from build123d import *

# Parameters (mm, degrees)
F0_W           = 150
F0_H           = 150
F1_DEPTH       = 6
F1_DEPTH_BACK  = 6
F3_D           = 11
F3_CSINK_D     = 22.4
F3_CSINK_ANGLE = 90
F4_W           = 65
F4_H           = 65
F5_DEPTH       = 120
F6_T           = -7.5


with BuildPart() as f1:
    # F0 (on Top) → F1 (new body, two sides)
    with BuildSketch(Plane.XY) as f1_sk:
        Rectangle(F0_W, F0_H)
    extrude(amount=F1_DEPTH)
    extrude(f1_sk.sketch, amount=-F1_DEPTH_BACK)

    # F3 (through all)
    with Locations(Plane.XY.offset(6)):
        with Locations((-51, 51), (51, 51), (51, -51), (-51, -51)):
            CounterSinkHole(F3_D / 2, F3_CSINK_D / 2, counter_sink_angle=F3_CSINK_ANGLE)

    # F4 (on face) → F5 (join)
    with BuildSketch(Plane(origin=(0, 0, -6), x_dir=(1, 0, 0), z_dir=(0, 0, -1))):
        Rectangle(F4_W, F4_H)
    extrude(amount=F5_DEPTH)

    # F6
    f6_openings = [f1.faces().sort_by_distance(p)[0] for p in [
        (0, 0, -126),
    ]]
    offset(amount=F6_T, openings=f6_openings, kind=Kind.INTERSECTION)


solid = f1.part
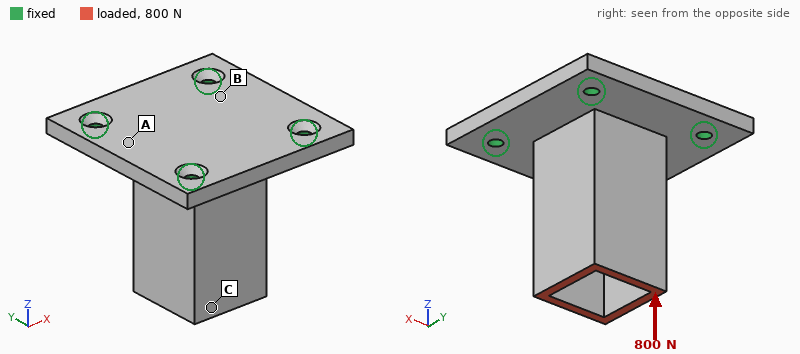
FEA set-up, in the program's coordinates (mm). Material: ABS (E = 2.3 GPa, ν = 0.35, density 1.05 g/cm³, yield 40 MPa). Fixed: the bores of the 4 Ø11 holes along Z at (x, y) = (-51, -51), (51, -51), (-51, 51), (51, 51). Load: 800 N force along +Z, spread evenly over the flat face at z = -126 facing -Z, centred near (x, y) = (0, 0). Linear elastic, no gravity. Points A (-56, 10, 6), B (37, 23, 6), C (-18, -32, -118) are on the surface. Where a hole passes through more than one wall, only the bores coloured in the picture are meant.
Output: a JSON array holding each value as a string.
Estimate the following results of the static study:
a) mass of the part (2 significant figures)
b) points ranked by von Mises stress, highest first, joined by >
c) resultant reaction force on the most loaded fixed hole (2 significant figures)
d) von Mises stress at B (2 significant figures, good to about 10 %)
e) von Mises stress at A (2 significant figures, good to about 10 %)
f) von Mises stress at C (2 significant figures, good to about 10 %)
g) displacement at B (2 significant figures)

["480 g", "B > A > C", "240 N", "1.6 MPa", "0.97 MPa", "0.46 MPa", "0.086 mm"]
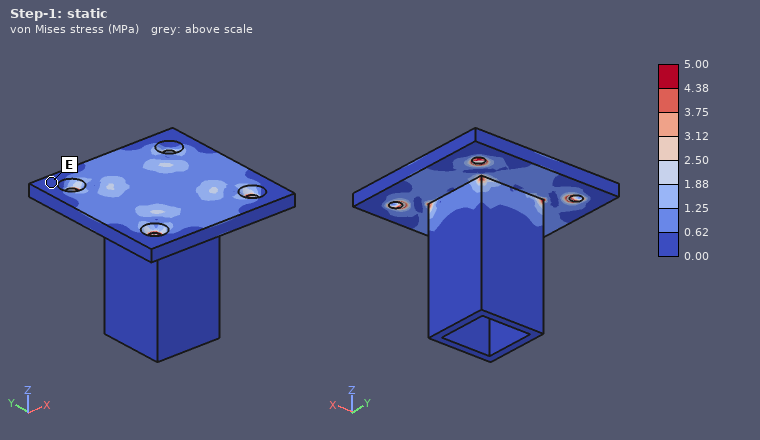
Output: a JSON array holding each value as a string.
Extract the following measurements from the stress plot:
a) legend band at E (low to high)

["0.00 to 0.62 MPa"]
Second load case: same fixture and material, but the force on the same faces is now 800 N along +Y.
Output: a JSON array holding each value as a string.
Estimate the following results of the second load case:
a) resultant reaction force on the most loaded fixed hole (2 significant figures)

["580 N"]
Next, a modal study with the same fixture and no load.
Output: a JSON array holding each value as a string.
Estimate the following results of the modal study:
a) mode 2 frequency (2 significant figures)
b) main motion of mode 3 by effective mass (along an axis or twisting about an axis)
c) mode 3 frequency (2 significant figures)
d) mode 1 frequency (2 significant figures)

["450 Hz", "along Z", "760 Hz", "450 Hz"]
